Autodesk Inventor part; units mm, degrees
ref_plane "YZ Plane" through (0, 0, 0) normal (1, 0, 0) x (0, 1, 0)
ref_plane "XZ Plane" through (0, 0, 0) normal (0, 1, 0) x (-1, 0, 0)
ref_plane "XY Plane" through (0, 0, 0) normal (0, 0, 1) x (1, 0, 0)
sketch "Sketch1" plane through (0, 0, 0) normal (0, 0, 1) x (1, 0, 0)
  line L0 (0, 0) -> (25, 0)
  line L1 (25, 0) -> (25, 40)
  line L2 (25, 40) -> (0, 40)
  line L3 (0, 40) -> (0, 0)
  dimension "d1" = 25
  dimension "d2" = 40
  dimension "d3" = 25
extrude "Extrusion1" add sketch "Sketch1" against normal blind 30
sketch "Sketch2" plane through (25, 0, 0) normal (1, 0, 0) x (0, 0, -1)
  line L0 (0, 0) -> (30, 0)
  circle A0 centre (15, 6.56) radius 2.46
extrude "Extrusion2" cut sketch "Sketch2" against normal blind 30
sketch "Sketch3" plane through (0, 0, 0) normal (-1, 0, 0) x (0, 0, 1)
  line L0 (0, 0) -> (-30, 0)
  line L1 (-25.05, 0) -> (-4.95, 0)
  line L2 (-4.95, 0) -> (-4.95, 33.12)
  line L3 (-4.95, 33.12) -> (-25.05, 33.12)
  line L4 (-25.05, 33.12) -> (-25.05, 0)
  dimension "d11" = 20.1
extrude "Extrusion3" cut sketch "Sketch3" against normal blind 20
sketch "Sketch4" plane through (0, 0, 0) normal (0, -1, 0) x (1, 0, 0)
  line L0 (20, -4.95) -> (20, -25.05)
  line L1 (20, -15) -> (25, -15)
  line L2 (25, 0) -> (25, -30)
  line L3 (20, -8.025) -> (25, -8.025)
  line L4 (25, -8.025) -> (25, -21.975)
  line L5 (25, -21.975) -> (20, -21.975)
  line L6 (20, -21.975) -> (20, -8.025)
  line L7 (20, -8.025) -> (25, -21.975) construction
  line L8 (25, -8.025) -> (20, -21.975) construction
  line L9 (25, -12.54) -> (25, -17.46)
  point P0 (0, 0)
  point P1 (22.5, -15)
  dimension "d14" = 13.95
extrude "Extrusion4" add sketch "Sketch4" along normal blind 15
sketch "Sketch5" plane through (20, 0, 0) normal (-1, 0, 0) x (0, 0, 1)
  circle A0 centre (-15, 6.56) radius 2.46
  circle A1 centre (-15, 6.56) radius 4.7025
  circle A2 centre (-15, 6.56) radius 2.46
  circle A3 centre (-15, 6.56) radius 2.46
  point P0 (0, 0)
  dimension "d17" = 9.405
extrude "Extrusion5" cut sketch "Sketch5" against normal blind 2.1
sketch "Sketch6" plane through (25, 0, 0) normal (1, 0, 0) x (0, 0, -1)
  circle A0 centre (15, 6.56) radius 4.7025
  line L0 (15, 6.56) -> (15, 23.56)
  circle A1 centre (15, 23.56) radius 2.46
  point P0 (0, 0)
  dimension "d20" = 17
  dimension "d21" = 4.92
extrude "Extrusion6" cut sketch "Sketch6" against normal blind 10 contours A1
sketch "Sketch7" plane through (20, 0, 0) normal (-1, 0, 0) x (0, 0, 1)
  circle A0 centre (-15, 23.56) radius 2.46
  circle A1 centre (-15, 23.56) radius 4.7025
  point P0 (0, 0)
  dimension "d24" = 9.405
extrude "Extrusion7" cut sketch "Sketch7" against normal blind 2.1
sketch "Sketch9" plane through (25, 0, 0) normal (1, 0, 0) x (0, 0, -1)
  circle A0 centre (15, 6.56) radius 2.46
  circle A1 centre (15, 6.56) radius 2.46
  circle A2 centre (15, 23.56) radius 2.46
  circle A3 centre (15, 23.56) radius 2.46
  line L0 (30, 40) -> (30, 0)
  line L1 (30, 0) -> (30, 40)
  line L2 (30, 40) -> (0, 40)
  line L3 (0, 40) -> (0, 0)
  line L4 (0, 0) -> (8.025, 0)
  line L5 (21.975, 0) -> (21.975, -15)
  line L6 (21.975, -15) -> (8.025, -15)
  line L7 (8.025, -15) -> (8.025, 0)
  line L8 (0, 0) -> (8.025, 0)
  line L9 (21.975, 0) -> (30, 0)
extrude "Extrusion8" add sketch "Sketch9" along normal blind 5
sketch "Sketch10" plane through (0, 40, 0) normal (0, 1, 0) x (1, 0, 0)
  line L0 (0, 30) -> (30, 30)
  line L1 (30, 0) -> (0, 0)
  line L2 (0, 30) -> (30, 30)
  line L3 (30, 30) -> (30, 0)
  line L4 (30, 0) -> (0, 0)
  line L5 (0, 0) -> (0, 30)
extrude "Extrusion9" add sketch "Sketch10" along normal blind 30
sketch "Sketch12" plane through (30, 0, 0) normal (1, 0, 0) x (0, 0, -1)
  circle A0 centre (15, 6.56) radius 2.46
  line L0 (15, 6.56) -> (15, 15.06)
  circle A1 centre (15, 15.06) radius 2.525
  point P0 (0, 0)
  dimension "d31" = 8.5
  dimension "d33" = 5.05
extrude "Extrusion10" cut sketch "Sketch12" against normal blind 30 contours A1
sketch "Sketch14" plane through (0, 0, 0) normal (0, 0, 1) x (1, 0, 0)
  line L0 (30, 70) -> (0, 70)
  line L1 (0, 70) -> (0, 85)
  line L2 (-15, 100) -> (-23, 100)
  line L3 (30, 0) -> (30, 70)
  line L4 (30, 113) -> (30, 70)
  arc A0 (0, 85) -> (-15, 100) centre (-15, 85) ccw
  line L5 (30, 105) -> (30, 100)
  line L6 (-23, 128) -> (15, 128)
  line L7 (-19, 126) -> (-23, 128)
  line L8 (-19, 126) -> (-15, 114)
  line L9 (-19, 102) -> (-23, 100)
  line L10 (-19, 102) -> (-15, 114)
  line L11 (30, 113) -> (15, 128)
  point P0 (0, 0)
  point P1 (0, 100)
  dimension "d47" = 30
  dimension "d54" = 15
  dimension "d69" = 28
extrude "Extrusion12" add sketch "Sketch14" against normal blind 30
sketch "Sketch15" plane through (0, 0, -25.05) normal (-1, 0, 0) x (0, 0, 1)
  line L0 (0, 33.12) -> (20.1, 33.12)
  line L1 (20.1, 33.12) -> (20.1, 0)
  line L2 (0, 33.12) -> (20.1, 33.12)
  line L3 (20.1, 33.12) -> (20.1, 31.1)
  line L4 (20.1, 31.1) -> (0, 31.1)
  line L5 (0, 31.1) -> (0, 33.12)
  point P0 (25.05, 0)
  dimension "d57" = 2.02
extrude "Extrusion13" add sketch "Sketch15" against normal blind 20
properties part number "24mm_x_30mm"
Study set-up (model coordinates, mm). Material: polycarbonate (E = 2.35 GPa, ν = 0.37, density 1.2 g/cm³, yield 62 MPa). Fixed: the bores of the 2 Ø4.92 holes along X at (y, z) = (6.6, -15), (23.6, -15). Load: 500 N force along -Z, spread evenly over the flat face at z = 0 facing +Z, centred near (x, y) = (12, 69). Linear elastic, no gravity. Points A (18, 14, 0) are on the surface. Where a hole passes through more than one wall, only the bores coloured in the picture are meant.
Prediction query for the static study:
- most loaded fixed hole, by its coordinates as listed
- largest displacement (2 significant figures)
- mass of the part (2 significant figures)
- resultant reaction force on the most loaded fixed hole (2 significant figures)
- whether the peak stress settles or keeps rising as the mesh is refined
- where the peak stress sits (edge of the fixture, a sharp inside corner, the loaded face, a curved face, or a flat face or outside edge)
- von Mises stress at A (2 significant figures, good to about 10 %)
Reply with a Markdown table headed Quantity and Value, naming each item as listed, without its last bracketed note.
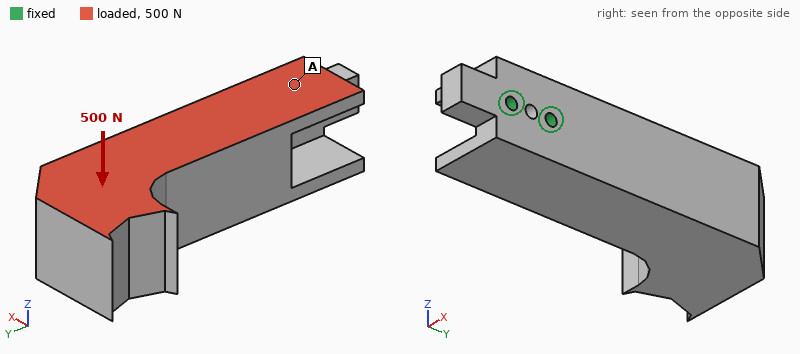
| Quantity | Value |
|---|---|
| most loaded fixed hole, by its coordinates as listed | (23.6, -15) |
| largest displacement | 1.7 mm |
| mass of the part | 140 g |
| resultant reaction force on the most loaded fixed hole | 1.5 kN |
| whether the peak stress settles or keeps rising as the mesh is refined | keeps rising |
| where the peak stress sits | edge of the fixture |
| von Mises stress at A | 5.2 MPa |
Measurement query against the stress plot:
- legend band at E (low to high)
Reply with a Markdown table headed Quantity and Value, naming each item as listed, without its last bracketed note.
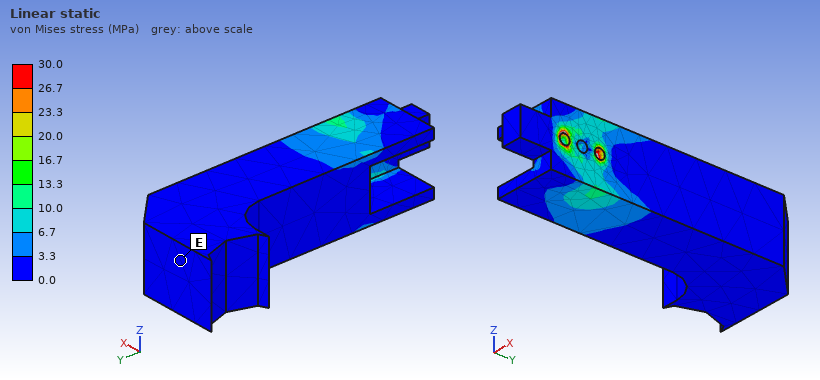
| Quantity | Value |
|---|---|
| legend band at E | 0.0 to 3.3 MPa |
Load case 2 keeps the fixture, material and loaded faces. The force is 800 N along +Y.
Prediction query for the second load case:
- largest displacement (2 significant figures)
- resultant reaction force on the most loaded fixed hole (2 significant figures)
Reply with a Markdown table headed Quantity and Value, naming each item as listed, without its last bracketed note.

| Quantity | Value |
|---|---|
| largest displacement | 1.2 mm |
| resultant reaction force on the most loaded fixed hole | 830 N |
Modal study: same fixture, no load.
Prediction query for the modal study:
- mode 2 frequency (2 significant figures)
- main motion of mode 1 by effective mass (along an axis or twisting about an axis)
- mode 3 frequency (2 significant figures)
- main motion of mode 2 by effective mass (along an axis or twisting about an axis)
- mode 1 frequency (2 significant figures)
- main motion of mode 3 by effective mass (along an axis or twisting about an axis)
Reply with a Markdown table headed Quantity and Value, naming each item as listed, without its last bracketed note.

| Quantity | Value |
|---|---|
| mode 2 frequency | 280 Hz |
| main motion of mode 1 by effective mass | along X |
| mode 3 frequency | 760 Hz |
| main motion of mode 2 by effective mass | along Z |
| mode 1 frequency | 240 Hz |
| main motion of mode 3 by effective mass | twisting about Y |
